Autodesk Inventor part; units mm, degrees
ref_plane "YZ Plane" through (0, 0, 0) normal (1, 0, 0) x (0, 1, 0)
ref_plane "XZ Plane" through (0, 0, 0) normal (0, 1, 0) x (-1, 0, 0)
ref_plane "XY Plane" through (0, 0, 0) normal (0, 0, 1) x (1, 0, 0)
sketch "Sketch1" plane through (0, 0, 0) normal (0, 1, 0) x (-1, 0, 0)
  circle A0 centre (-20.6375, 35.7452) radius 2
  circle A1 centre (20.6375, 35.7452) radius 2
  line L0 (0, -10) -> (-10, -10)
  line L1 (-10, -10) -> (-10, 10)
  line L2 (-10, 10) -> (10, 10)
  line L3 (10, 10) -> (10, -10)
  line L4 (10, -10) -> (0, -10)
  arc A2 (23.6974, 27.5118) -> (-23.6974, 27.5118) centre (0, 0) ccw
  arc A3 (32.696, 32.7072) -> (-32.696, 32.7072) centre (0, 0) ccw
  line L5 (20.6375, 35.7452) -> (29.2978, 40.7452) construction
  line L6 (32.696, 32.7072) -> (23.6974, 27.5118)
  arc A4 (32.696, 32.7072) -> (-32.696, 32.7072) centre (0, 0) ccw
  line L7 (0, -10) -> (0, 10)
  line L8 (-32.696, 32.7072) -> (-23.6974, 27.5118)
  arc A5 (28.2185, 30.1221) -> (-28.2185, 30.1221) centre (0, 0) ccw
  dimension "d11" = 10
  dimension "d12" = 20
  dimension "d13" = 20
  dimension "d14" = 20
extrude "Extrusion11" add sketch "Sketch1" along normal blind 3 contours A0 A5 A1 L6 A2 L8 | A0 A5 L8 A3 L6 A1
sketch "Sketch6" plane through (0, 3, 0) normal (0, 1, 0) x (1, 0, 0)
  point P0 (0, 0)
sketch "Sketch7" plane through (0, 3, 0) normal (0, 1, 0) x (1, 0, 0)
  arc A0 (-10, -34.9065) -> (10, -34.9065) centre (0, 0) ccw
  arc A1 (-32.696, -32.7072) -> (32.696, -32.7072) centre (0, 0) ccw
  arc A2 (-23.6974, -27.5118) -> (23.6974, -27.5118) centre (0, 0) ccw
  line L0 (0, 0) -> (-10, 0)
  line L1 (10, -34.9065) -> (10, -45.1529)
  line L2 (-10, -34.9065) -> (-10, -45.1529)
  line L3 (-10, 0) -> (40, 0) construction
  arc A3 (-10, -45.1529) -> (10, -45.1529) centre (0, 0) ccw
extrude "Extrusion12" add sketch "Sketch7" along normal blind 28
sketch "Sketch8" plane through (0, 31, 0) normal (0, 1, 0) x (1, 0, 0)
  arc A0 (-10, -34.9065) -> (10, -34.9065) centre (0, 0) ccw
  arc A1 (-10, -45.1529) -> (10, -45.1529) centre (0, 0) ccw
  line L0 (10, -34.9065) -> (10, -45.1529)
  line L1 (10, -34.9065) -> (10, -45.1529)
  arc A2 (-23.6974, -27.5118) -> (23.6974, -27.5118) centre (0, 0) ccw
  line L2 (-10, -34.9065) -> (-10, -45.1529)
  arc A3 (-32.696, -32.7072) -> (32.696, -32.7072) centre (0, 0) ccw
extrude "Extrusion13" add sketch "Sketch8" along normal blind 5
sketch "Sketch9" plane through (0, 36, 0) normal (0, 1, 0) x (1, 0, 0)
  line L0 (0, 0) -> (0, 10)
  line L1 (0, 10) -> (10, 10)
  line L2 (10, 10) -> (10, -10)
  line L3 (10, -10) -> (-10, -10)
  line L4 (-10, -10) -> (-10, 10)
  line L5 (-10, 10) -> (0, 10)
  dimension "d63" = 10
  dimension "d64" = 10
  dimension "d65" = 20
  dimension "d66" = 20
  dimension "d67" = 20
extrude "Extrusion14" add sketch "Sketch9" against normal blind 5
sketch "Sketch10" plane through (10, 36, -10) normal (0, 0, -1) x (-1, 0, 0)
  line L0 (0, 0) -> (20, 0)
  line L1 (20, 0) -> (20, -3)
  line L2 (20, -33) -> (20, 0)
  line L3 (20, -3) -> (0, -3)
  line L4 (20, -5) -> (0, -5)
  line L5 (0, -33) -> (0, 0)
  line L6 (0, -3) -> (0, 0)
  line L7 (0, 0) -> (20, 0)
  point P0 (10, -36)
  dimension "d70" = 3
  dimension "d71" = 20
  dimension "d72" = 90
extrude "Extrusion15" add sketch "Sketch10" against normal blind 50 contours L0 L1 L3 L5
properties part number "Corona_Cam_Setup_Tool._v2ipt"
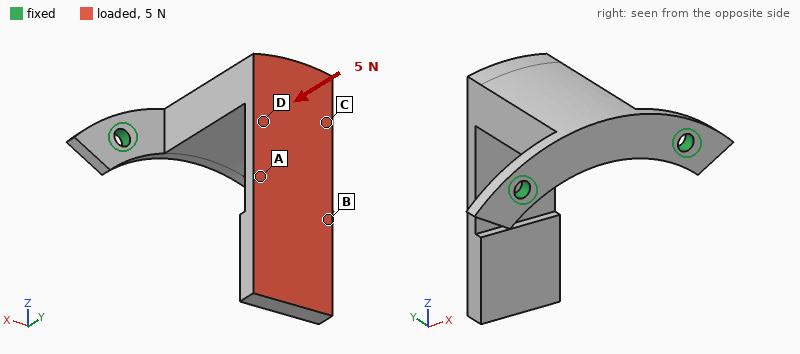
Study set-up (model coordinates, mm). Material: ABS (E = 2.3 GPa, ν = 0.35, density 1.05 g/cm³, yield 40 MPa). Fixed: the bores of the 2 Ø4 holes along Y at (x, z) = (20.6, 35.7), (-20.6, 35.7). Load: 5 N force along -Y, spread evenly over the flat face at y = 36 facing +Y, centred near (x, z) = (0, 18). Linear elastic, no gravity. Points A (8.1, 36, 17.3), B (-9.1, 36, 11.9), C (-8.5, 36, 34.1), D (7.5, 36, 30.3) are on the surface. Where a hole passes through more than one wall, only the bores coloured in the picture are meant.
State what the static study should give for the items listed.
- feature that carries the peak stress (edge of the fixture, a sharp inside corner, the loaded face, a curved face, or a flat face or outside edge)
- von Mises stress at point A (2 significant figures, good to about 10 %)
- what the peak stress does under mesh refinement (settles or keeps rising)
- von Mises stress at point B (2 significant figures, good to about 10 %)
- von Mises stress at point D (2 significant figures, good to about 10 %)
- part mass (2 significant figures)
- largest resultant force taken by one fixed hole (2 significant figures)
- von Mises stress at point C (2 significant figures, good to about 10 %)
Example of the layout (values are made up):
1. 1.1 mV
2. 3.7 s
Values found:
1. edge of the fixture
2. 1.2 MPa
3. keeps rising
4. 0.71 MPa
5. 2.4 MPa
6. 13 g
7. 3.1 N
8. 2.8 MPa
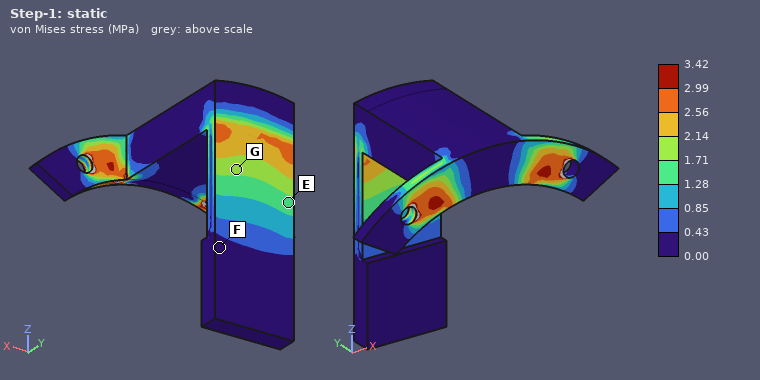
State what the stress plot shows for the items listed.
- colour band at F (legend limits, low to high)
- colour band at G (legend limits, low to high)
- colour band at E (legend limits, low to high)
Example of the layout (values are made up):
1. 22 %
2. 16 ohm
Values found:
1. 0.00 to 0.43 MPa
2. 1.71 to 2.14 MPa
3. 1.28 to 1.71 MPa
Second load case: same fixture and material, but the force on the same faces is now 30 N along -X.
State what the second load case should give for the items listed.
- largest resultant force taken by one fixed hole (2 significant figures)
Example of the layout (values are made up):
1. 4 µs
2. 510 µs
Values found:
1. 41 N
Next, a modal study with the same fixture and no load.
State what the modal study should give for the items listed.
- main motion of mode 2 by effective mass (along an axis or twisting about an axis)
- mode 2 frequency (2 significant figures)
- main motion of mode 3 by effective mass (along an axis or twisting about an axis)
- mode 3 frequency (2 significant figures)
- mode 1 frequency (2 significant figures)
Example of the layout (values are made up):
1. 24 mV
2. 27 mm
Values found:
1. along Z
2. 340 Hz
3. along X
4. 520 Hz
5. 160 Hz
